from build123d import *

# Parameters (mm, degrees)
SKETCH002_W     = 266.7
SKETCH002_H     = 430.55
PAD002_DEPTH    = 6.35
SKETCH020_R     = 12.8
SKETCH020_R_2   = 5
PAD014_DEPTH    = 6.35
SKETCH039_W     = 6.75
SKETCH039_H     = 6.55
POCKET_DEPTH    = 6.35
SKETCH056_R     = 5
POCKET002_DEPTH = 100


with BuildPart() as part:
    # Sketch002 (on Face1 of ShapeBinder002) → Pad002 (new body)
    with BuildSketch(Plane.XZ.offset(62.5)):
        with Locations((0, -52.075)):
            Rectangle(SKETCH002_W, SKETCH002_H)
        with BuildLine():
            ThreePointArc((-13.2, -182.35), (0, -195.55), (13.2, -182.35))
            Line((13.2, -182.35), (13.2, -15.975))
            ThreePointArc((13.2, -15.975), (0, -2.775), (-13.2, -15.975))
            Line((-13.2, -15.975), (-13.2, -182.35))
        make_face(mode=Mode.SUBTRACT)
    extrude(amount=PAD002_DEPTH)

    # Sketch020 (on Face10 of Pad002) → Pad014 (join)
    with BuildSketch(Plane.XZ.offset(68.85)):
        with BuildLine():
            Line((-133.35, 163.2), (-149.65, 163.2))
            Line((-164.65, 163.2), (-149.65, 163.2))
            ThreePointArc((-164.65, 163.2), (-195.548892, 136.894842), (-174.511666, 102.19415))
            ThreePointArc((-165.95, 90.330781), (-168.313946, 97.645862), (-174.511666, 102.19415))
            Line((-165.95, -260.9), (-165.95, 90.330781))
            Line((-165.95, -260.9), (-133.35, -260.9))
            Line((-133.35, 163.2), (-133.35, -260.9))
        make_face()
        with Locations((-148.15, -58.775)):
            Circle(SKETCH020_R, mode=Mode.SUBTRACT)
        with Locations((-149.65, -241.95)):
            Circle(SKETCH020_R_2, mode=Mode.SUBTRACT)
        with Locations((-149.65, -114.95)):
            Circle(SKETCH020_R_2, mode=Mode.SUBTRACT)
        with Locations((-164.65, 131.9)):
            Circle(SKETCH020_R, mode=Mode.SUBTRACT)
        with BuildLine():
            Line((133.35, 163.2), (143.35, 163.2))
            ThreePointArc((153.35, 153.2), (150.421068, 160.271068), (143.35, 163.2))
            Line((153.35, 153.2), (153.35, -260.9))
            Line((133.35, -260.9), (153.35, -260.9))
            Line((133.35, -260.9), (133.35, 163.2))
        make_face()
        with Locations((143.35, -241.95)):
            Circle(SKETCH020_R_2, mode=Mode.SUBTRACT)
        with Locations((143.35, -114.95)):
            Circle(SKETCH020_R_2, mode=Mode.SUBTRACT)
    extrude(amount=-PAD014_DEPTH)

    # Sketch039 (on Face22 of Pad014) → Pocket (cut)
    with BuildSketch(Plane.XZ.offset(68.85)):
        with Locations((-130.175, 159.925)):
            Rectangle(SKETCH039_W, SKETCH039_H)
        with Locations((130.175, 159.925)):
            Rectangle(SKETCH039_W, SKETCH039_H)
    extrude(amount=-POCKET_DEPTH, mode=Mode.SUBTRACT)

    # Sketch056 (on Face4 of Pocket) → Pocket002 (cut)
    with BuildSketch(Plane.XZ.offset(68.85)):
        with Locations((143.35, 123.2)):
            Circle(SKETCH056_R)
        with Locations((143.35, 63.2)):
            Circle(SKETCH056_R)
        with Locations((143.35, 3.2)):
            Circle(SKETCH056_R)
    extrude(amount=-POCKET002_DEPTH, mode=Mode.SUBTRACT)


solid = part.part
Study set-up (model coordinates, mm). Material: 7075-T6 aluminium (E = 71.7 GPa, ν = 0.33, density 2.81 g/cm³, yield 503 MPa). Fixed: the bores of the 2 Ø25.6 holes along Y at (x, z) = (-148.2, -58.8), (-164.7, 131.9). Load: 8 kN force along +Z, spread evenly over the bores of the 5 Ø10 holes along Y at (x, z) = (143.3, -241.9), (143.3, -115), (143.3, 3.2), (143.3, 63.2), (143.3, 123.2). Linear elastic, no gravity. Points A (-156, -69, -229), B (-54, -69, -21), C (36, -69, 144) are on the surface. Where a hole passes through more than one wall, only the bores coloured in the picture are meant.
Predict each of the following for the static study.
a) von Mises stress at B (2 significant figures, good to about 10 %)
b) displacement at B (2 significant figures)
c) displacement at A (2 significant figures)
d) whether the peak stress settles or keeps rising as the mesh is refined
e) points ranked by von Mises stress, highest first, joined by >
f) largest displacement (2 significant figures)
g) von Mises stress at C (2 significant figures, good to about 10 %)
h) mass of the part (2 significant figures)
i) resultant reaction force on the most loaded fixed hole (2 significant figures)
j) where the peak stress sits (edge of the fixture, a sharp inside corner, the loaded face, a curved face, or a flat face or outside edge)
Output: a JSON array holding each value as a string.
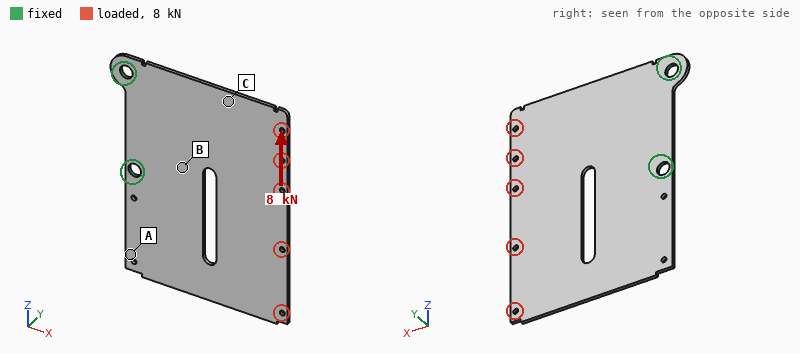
["23 MPa", "0.051 mm", "0.14 mm", "keeps rising", "B > C > A", "0.27 mm", "9.8 MPa", "2.4 kg", "12 kN", "edge of the fixture"]
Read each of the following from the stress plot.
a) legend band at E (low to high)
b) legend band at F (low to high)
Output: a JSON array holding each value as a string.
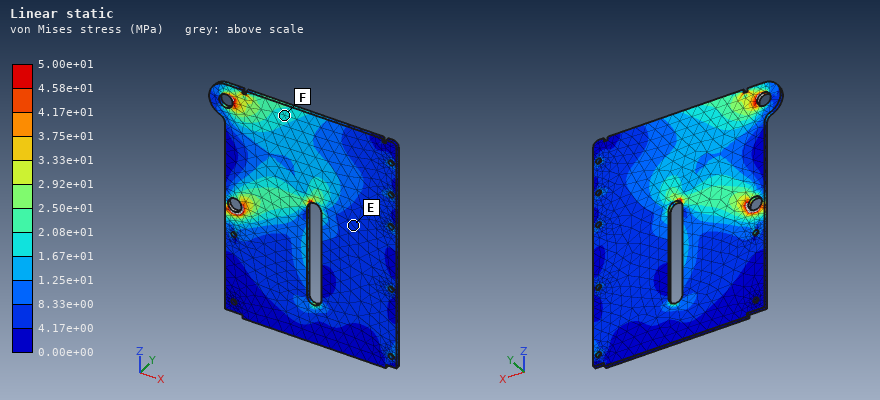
["4.17e+00 to 8.33e+00 MPa", "1.67e+01 to 2.08e+01 MPa"]
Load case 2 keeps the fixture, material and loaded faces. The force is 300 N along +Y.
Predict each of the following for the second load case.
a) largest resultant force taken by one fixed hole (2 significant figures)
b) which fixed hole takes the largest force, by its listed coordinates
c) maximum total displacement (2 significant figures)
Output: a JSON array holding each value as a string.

["290 N", "(-148.2, -58.8)", "6.3 mm"]
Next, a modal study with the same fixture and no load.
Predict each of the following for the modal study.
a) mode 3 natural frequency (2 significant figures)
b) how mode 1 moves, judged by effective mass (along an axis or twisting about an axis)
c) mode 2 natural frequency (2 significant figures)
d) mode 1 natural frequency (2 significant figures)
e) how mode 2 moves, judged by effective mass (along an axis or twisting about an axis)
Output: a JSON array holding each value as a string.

["160 Hz", "along Y", "76 Hz", "45 Hz", "twisting about X"]
